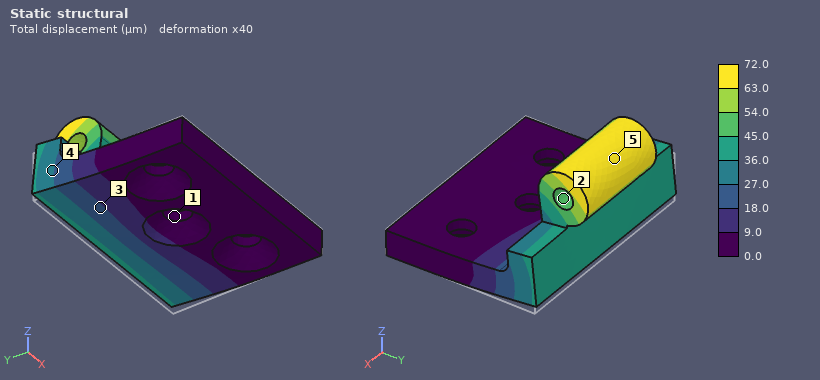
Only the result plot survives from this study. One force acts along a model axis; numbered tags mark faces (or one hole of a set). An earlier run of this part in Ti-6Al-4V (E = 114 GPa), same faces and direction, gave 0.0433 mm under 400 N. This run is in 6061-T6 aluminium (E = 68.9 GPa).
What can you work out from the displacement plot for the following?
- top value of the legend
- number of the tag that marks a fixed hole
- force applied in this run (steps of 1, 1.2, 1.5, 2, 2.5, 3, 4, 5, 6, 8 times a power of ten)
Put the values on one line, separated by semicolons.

72.0 µm; 1; 400 N
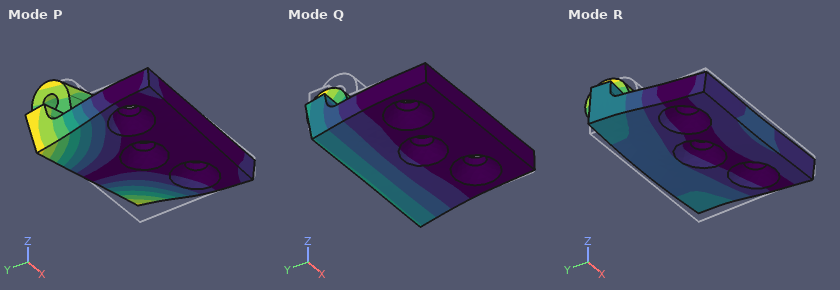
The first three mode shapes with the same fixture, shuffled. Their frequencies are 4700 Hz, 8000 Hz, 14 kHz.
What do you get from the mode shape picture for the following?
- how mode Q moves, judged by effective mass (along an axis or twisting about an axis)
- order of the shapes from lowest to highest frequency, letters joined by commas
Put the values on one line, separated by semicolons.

along Z; Q, P, R
